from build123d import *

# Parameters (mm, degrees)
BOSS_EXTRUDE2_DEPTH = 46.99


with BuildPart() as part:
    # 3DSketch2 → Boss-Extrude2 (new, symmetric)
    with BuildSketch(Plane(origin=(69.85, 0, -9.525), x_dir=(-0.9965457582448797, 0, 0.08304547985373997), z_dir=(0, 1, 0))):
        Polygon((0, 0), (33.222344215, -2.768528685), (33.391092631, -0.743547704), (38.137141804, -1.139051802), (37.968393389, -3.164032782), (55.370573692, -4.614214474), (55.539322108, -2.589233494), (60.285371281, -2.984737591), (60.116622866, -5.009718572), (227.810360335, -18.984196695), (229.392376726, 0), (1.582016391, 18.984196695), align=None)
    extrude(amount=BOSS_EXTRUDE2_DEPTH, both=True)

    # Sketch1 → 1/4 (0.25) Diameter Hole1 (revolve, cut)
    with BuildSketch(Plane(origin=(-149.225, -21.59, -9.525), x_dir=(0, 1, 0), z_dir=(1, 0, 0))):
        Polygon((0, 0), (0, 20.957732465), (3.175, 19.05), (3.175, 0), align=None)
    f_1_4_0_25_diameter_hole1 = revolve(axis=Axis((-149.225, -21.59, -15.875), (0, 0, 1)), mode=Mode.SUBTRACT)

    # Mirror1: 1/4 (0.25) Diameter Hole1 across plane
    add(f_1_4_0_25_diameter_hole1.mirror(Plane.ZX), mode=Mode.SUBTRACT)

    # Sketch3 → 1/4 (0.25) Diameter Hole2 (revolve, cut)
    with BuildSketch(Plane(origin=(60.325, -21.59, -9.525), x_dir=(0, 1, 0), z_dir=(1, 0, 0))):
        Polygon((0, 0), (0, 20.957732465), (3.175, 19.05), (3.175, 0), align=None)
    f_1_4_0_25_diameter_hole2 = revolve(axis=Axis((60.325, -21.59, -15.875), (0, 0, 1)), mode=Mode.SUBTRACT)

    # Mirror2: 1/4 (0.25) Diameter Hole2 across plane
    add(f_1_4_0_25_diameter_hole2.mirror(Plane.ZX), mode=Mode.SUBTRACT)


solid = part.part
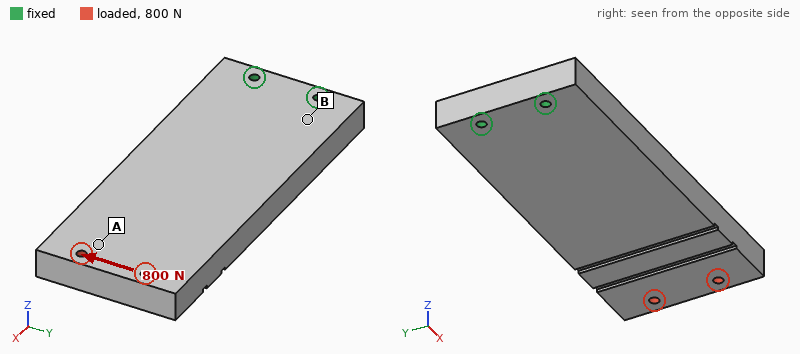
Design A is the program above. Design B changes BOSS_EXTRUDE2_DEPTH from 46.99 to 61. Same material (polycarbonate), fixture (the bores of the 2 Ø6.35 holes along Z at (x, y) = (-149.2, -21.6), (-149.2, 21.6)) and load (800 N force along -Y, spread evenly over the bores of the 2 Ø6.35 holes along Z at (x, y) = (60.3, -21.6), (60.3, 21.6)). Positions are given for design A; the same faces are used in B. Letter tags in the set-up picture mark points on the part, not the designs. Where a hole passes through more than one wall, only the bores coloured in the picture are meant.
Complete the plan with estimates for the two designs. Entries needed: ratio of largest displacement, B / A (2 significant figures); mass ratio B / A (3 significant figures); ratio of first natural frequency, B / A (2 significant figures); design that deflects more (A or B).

0.83
1.30
0.95
A
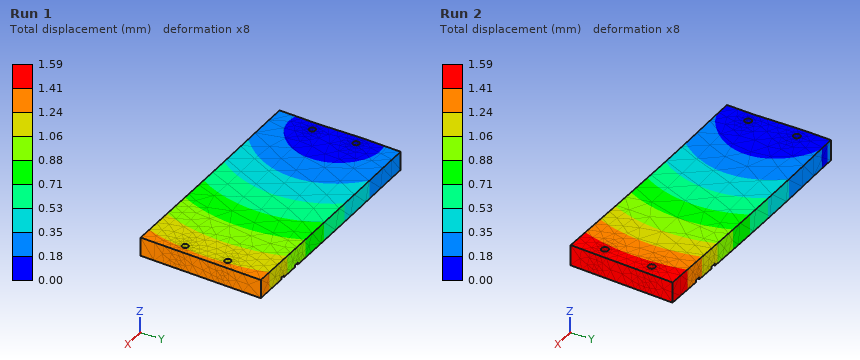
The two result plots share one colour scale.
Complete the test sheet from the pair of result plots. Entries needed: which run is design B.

Run 1
